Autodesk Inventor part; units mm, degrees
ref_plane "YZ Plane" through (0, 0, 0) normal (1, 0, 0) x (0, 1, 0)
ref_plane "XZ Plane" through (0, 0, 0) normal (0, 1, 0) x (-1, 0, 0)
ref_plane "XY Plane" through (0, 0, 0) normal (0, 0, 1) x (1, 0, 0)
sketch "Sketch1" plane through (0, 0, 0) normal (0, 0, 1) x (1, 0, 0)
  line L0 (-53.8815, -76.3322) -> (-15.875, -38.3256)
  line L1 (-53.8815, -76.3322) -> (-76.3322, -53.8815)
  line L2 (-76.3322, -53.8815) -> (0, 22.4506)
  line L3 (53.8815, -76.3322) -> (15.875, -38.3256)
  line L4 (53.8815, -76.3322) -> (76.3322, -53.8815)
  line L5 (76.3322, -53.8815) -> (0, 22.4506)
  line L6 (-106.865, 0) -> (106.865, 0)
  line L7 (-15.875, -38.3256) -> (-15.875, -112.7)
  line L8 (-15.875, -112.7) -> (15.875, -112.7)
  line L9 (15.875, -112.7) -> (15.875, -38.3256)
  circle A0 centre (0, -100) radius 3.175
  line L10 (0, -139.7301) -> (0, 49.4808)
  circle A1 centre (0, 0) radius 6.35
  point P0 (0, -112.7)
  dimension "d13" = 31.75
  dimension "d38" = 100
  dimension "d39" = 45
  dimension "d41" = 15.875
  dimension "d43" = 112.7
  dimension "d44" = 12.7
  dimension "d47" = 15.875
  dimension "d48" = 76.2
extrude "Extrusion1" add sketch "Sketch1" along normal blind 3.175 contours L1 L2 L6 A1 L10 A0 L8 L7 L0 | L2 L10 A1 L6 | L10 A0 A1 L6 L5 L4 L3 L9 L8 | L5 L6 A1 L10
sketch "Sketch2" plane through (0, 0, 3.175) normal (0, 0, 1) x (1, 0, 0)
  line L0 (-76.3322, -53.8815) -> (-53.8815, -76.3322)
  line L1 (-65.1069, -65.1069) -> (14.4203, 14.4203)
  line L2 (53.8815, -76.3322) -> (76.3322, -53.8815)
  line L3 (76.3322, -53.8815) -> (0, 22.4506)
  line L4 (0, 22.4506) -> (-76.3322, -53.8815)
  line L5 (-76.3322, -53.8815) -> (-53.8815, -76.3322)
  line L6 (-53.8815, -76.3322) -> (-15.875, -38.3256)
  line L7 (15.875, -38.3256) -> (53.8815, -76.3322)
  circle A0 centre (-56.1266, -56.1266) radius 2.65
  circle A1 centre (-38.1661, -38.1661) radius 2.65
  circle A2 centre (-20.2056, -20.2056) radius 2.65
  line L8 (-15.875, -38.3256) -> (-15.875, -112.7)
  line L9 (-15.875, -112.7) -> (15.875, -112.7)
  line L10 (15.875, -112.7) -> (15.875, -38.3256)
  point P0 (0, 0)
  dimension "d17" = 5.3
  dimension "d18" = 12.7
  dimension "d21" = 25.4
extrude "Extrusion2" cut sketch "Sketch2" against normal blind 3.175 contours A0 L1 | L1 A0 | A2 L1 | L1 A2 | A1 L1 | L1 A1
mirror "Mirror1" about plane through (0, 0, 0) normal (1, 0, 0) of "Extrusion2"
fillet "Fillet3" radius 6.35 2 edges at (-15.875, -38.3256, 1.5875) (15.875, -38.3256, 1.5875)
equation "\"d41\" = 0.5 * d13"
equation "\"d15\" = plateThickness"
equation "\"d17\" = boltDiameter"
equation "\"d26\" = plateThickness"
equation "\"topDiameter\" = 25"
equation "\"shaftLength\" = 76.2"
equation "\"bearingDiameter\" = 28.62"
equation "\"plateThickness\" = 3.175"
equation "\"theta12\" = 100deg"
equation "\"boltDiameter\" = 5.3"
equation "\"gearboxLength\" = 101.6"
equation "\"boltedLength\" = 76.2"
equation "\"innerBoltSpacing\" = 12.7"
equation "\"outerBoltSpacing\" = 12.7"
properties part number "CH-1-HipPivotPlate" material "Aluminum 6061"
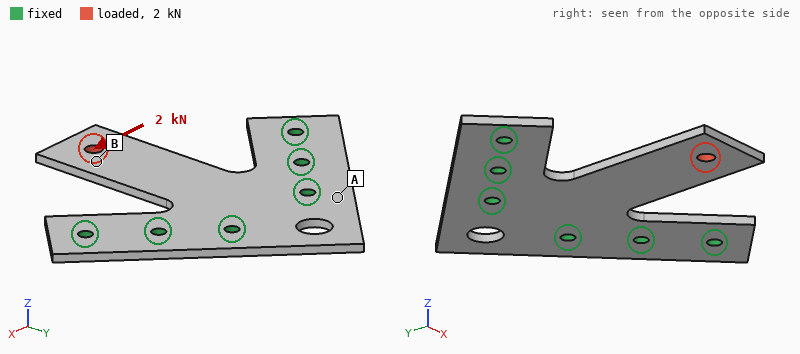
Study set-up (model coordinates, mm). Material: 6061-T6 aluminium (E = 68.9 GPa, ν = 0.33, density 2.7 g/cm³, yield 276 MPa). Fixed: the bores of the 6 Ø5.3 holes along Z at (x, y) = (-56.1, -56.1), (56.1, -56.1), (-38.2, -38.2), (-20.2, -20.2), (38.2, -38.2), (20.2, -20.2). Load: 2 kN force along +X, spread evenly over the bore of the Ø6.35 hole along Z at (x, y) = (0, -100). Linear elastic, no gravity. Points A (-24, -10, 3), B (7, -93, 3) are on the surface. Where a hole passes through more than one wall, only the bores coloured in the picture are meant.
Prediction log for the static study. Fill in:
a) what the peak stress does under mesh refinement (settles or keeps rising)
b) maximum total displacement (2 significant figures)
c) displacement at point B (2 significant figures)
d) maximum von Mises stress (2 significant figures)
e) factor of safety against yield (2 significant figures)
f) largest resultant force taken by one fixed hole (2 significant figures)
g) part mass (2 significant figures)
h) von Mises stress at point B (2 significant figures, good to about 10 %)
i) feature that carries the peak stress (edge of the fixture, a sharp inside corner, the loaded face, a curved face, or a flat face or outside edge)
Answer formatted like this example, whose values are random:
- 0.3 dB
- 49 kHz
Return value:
- settles
- 0.38 mm
- 0.24 mm
- 310 MPa
- 0.90
- 1.8 kN
- 71 g
- 40 MPa
- a curved face
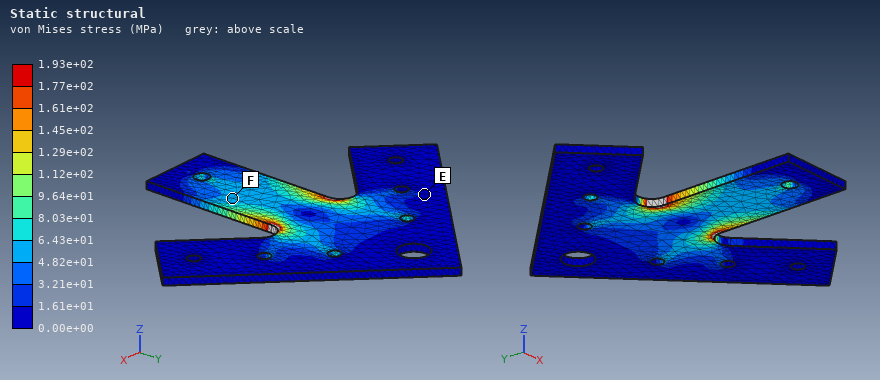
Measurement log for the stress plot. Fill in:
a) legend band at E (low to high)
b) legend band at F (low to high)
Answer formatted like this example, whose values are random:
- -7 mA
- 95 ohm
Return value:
- 0.00e+00 to 1.61e+01 MPa
- 4.82e+01 to 6.43e+01 MPa
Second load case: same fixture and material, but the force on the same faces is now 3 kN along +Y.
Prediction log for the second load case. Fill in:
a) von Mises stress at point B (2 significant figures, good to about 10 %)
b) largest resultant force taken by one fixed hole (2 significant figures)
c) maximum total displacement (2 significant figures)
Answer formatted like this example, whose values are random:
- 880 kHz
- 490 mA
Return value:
- 36 MPa
- 1.3 kN
- 40 µm
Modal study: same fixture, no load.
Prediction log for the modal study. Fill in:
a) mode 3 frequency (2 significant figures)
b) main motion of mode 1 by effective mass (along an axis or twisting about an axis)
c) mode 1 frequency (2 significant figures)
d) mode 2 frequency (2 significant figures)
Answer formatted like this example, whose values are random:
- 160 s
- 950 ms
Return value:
- 2300 Hz
- along Z
- 430 Hz
- 2200 Hz
